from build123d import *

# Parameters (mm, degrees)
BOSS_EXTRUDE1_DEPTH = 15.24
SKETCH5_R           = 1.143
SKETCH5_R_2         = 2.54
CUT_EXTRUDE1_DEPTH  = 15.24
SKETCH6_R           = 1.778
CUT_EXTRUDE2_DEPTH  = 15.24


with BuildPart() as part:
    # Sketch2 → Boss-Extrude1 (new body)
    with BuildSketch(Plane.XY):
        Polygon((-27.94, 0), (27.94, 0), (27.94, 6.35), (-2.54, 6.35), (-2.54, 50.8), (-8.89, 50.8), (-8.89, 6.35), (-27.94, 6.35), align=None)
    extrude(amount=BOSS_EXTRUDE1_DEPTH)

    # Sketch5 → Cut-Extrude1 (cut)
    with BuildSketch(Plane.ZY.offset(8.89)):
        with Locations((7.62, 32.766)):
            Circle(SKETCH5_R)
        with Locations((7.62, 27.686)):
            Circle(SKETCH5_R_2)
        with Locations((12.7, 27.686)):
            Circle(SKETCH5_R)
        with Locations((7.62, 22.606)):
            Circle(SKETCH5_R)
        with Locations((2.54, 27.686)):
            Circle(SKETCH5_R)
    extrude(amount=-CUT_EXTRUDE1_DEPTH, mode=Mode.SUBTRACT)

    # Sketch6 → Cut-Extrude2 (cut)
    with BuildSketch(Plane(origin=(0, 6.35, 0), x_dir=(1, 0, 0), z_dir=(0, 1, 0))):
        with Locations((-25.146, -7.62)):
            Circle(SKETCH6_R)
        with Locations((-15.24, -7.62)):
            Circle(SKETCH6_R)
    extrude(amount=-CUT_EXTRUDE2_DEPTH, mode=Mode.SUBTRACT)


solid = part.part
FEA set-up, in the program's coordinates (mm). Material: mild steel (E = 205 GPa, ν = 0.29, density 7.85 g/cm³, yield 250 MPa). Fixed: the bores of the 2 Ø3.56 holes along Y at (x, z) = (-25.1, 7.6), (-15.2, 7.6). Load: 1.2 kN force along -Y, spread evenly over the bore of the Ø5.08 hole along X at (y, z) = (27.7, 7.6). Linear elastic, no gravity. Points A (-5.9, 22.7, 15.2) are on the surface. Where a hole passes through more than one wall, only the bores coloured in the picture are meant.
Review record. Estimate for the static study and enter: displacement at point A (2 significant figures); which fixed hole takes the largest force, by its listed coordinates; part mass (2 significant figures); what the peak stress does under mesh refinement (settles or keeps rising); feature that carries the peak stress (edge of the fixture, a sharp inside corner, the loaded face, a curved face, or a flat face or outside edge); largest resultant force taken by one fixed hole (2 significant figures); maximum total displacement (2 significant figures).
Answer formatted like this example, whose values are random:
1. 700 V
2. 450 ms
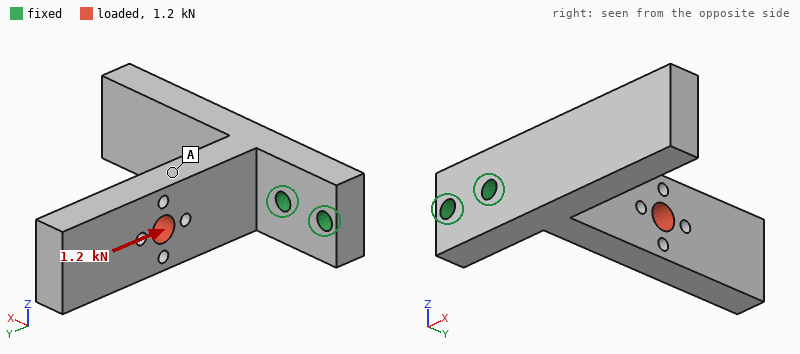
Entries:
1. 19 µm
2. (-15.2, 7.6)
3. 73 g
4. keeps rising
5. edge of the fixture
6. 1.4 kN
7. 44 µm
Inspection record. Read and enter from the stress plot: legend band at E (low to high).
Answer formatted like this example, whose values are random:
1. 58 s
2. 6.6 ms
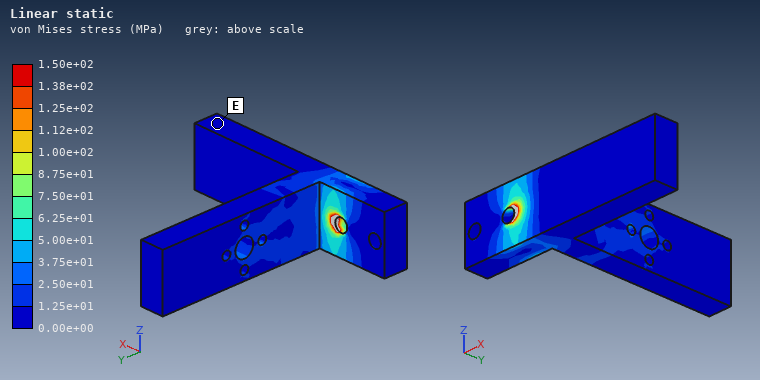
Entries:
1. 0.00e+00 to 1.25e+01 MPa
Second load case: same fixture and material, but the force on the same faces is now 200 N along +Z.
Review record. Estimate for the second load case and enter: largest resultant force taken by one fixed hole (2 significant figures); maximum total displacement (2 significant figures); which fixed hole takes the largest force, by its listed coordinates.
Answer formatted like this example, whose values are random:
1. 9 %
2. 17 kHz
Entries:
1. 310 N
2. 28 µm
3. (-15.2, 7.6)
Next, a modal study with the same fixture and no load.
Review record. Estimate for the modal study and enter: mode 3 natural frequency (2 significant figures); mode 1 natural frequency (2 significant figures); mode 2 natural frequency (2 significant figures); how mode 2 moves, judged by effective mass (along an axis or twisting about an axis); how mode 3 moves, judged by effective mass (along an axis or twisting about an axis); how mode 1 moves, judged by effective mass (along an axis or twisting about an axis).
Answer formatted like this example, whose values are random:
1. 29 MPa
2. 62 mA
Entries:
1. 3600 Hz
2. 1700 Hz
3. 2700 Hz
4. along Z
5. along Y
6. along X
